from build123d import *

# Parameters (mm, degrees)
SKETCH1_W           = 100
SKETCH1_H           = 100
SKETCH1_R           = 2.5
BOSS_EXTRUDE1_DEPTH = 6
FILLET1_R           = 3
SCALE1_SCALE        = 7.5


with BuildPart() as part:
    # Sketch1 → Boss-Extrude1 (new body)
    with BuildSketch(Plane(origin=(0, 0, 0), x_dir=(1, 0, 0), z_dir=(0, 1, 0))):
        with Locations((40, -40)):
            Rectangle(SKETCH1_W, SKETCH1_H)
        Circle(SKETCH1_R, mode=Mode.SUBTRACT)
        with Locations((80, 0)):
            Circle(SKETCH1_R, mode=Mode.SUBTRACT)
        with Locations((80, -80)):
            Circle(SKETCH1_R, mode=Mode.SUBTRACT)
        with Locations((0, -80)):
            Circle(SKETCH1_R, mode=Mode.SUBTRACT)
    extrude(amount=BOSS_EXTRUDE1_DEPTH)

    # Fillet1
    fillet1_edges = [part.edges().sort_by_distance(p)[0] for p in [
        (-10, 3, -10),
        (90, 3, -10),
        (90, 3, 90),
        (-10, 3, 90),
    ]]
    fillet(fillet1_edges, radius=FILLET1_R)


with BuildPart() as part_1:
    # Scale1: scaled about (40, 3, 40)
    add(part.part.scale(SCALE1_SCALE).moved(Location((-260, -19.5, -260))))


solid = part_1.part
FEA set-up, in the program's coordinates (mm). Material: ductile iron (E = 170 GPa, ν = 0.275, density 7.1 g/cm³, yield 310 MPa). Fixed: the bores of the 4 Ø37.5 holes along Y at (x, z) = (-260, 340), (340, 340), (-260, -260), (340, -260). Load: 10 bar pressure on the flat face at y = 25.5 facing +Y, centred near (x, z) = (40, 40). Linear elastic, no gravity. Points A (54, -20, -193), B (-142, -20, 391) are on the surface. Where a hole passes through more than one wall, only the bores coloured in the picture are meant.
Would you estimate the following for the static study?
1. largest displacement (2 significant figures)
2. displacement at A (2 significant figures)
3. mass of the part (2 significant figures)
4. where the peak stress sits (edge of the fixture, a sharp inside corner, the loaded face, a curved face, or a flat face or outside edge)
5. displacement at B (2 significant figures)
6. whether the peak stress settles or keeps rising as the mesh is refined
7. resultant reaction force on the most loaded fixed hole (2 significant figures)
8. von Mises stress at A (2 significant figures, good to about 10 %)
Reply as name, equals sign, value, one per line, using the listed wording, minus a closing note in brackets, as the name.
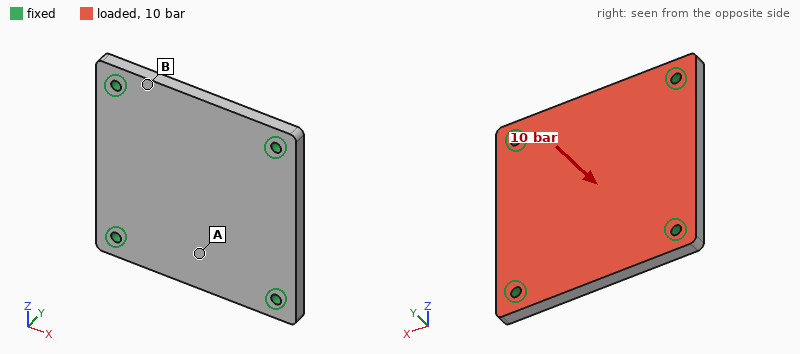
largest displacement = 0.73 mm
displacement at A = 0.50 mm
mass of the part = 180 kg
where the peak stress sits = edge of the fixture
displacement at B = 0.13 mm
whether the peak stress settles or keeps rising as the mesh is refined = keeps rising
resultant reaction force on the most loaded fixed hole = 140 kN
von Mises stress at A = 54 MPa
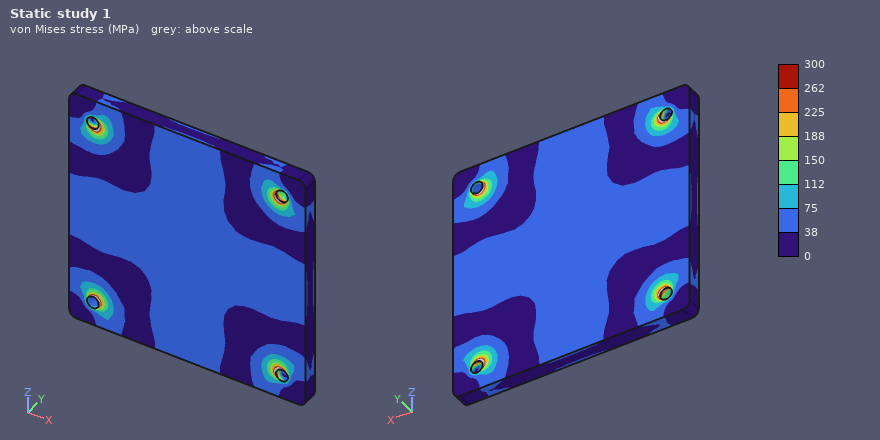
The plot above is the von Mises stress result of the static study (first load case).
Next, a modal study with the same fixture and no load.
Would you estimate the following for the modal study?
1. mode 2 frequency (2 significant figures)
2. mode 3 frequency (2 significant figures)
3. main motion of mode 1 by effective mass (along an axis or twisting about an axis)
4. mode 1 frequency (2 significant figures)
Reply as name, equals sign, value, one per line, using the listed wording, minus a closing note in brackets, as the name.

mode 2 frequency = 660 Hz
mode 3 frequency = 660 Hz
main motion of mode 1 by effective mass = along Y
mode 1 frequency = 400 Hz
